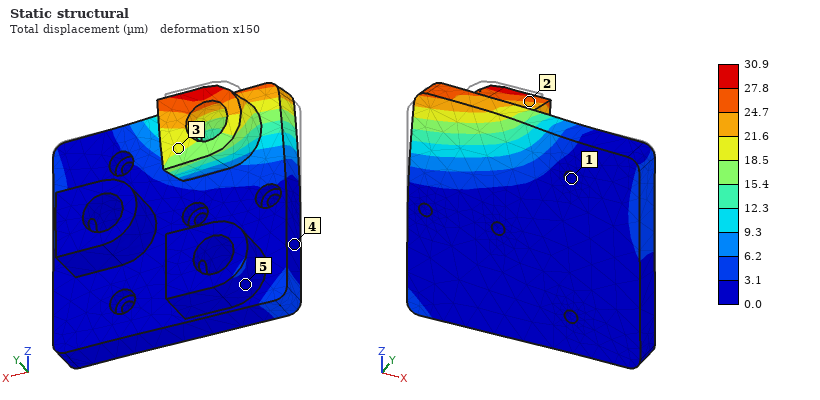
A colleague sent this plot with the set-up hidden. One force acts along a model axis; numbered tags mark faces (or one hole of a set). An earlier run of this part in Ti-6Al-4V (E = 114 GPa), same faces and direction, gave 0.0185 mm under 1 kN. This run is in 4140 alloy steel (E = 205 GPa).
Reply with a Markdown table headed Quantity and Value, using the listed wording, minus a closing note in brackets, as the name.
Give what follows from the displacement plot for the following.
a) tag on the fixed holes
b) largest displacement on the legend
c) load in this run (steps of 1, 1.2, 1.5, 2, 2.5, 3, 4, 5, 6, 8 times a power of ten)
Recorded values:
| Quantity | Value |
|---|---|
| tag on the fixed holes | 1 |
| largest displacement on the legend | 30.9 µm |
| load in this run | 3 kN |
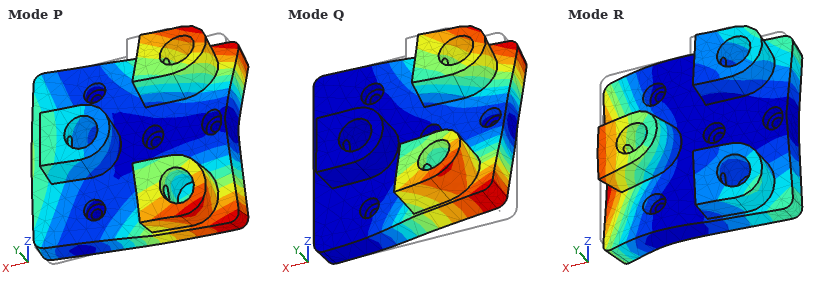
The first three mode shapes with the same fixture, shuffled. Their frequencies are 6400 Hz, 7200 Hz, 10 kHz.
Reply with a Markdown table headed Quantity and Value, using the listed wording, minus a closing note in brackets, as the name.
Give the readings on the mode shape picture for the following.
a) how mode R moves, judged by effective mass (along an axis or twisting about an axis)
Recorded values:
| Quantity | Value |
|---|---|
| how mode R moves, judged by effective mass | along Y |
